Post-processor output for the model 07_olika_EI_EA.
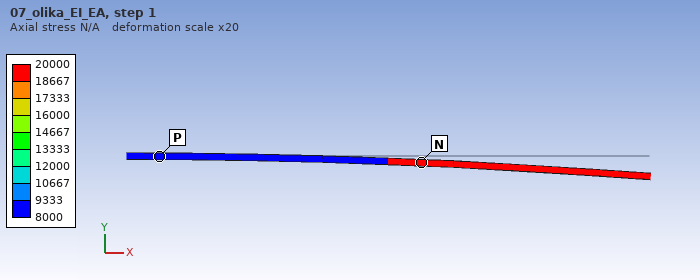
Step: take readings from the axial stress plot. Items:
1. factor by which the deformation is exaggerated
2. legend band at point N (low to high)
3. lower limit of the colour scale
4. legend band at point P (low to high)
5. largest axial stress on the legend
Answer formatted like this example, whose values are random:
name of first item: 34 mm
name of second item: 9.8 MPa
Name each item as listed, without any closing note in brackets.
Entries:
factor by which the deformation is exaggerated: 20
legend band at point N: 18667 to 20000
lower limit of the colour scale: 8000
legend band at point P: 8000 to 9333
largest axial stress on the legend: 20000
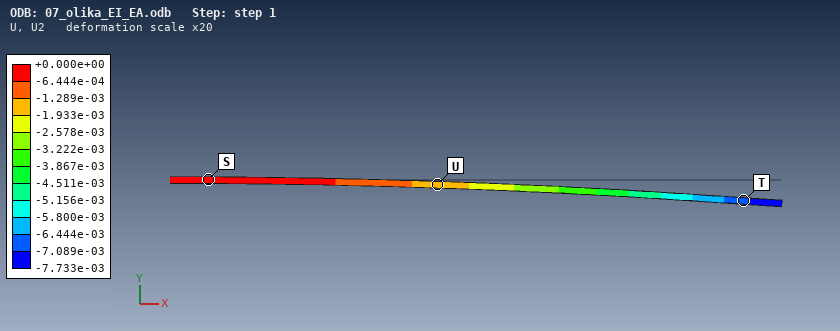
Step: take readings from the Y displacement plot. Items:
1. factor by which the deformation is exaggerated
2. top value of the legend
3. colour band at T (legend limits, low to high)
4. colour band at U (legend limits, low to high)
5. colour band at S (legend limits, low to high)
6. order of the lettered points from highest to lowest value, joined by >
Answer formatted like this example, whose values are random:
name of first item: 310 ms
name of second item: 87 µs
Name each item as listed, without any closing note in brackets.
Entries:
factor by which the deformation is exaggerated: 20
top value of the legend: +0.000e+00
colour band at T: -7.089e-03 to -6.444e-03
colour band at U: -1.933e-03 to -1.289e-03
colour band at S: -6.444e-04 to +0.000e+00
order of the lettered points from highest to lowest value, joined by >: S > U > T
